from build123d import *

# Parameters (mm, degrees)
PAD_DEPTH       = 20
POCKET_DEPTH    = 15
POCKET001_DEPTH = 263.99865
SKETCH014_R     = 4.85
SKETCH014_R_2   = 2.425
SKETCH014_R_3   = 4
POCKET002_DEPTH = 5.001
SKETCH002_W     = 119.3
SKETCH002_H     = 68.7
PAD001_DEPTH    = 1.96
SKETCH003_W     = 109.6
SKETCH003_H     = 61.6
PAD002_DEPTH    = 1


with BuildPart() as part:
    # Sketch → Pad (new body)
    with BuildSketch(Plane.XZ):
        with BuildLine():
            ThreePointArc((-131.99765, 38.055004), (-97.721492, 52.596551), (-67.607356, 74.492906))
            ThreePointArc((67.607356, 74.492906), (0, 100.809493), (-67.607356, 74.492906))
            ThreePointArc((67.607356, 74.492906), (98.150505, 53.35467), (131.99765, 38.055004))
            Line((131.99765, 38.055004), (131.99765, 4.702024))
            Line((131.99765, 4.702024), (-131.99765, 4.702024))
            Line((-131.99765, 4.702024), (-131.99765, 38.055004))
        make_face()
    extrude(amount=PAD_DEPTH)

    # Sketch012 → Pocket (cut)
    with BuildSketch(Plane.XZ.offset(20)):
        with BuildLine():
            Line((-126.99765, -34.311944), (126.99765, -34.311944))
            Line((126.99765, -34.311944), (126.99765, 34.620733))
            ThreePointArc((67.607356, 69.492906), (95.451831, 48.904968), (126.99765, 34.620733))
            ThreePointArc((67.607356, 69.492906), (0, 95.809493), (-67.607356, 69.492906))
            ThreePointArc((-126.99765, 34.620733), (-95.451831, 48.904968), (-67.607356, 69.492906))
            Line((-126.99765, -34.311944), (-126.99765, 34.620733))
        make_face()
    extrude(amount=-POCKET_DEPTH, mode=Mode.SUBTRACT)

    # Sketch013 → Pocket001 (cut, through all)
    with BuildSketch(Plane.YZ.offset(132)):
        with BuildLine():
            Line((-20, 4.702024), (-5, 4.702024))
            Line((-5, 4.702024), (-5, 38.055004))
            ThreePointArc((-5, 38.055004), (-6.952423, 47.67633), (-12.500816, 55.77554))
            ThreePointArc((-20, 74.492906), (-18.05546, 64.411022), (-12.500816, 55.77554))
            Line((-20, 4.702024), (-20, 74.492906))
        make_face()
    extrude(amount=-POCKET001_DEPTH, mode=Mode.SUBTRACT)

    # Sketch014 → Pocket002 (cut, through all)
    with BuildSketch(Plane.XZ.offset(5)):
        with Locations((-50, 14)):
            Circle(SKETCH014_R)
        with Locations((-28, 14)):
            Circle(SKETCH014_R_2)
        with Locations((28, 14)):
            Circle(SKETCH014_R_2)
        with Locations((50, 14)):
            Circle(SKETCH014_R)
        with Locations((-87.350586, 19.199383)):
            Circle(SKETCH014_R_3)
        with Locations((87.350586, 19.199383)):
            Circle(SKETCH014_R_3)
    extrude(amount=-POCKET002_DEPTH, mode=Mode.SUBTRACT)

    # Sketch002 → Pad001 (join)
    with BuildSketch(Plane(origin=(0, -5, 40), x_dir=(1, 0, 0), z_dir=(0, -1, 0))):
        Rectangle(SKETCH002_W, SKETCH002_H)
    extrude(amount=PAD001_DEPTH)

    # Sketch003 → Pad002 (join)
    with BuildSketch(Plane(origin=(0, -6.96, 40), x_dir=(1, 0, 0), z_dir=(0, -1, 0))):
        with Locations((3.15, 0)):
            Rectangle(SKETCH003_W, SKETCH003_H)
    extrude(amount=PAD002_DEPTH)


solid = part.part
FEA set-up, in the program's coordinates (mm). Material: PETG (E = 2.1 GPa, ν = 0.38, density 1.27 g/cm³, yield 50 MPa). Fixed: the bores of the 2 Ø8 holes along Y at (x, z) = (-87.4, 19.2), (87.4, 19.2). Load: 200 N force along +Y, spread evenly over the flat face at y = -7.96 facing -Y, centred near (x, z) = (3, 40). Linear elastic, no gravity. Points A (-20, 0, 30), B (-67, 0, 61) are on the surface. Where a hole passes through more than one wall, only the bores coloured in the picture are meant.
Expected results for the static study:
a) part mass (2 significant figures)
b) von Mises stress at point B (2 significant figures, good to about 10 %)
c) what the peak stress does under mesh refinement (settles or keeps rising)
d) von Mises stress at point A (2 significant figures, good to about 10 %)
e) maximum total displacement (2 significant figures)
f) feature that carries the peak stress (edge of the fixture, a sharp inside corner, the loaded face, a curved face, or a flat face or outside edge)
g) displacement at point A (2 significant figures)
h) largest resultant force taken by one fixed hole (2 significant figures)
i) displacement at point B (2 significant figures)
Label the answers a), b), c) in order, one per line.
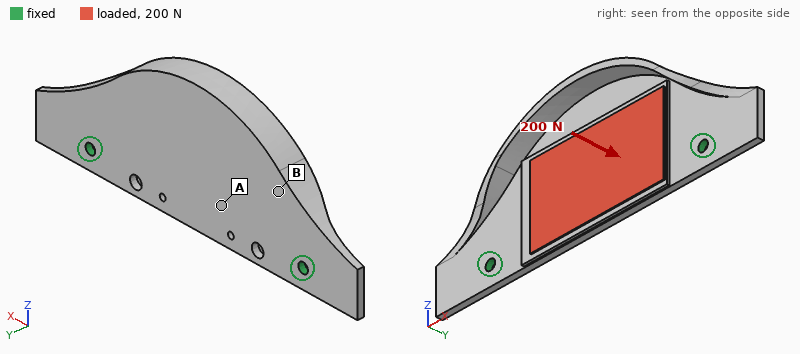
a) 160 g
b) 1.5 MPa
c) keeps rising
d) 2.6 MPa
e) 2.8 mm
f) edge of the fixture
g) 1.1 mm
h) 150 N
i) 1.1 mm
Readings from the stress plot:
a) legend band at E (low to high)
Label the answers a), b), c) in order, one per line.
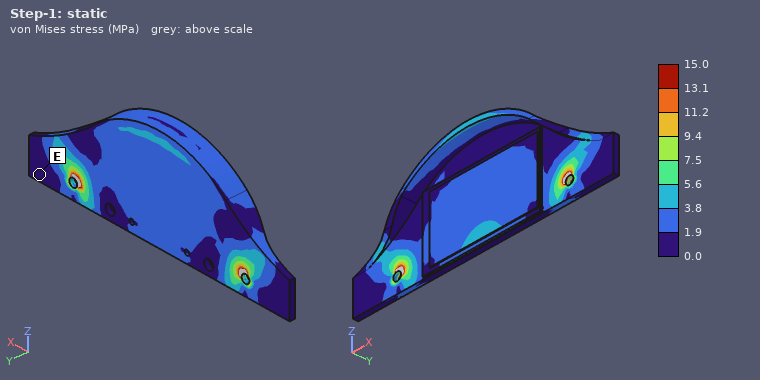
a) 0.0 to 1.9 MPa
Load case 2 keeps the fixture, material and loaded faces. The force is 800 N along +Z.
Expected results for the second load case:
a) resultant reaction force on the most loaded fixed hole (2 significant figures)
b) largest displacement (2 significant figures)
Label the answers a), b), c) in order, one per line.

a) 500 N
b) 3.1 mm
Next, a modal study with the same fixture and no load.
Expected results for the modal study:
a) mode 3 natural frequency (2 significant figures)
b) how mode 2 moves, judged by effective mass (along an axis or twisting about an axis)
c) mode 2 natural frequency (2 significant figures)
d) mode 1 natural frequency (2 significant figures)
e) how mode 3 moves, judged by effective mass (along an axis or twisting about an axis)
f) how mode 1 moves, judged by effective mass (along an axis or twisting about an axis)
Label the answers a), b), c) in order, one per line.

a) 490 Hz
b) along Y
c) 320 Hz
d) 120 Hz
e) twisting about Z
f) along Y
